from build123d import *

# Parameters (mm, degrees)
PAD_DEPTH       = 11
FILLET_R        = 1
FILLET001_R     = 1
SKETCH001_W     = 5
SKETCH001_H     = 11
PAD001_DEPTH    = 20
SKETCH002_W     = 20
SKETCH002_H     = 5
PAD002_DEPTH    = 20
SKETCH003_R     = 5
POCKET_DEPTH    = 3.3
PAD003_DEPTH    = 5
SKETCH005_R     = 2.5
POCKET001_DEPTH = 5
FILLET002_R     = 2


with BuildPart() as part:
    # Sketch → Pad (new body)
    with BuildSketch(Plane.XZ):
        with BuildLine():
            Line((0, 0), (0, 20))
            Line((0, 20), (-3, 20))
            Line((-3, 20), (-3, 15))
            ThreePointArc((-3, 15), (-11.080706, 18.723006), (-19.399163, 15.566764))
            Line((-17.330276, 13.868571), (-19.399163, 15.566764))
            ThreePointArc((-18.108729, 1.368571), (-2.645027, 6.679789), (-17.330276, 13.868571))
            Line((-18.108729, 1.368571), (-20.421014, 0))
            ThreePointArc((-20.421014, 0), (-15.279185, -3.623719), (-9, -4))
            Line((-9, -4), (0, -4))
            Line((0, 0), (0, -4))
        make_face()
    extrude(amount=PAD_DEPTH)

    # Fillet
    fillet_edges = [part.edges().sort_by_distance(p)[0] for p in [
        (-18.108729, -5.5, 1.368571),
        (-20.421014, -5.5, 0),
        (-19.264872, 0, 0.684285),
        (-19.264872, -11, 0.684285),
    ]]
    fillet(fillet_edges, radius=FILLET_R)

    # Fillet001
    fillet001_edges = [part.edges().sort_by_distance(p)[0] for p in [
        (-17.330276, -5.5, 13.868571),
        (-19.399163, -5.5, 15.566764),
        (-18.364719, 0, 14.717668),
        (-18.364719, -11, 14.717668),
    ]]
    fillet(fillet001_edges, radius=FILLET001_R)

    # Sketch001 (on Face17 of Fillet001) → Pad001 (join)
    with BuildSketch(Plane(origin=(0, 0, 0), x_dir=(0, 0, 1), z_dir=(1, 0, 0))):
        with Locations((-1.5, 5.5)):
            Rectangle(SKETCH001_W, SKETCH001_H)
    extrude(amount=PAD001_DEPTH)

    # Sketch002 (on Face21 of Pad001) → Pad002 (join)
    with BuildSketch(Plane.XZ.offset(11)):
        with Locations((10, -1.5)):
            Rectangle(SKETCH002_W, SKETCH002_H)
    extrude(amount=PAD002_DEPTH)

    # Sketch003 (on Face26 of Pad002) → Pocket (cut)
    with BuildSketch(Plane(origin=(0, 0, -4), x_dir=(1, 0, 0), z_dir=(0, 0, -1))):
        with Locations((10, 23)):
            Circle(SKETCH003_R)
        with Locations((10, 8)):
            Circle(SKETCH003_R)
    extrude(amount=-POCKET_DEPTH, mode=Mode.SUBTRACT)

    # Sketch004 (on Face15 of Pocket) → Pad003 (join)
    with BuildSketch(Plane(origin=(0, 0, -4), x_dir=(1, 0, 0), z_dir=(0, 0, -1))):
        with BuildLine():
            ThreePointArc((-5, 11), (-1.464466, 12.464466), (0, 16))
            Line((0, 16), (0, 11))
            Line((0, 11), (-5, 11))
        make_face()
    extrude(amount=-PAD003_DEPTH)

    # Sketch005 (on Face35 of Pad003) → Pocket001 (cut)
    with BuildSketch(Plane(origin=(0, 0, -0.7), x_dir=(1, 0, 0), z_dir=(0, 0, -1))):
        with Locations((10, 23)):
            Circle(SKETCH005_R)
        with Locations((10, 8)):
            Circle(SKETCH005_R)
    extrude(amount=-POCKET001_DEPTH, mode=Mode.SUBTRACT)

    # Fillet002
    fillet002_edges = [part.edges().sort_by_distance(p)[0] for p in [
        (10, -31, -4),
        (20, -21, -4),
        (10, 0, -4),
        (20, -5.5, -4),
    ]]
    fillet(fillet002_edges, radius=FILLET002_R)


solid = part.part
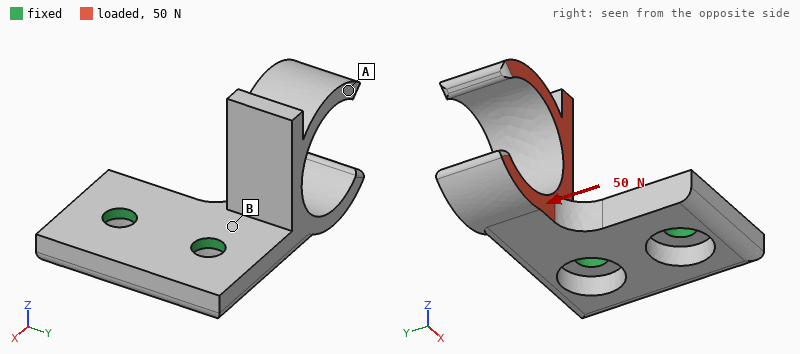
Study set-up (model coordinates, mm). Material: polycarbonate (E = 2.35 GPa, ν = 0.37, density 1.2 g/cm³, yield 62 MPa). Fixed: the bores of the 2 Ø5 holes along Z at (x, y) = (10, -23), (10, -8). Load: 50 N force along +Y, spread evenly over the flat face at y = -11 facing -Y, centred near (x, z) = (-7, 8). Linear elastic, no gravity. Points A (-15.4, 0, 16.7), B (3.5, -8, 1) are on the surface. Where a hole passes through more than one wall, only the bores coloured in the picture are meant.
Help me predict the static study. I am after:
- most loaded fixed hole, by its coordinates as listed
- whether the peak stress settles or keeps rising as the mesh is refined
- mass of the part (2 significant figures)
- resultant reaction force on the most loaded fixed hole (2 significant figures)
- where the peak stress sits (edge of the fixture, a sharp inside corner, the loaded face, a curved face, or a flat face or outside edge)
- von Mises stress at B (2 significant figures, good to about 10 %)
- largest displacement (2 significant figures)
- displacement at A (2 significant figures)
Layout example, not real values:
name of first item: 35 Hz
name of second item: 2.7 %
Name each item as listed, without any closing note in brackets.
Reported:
most loaded fixed hole, by its coordinates as listed: (10, -8)
whether the peak stress settles or keeps rising as the mesh is refined: keeps rising
mass of the part: 5.3 g
resultant reaction force on the most loaded fixed hole: 63 N
where the peak stress sits: a sharp inside corner
von Mises stress at B: 7.3 MPa
largest displacement: 0.66 mm
displacement at A: 0.61 mm
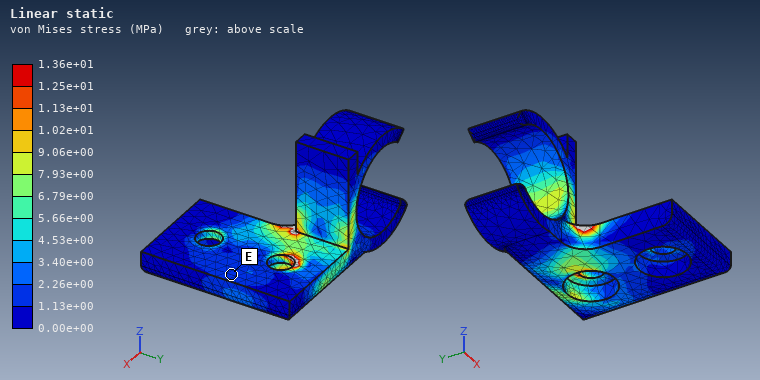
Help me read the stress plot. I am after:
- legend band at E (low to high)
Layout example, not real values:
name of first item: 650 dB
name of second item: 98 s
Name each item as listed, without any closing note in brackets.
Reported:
legend band at E: 1.13e+00 to 2.26e+00 MPa
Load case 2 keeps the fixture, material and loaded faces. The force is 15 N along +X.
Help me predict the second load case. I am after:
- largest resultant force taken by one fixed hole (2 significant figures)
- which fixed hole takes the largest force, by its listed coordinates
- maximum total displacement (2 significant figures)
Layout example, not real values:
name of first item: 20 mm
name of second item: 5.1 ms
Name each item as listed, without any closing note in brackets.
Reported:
largest resultant force taken by one fixed hole: 14 N
which fixed hole takes the largest force, by its listed coordinates: (10, -8)
maximum total displacement: 0.52 mm
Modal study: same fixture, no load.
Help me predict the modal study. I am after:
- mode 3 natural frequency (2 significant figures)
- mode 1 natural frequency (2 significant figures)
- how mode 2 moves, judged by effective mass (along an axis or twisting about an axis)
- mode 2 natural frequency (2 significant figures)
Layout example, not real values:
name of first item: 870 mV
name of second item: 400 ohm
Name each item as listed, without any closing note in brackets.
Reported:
mode 3 natural frequency: 1600 Hz
mode 1 natural frequency: 630 Hz
how mode 2 moves, judged by effective mass: along Y
mode 2 natural frequency: 1200 Hz
